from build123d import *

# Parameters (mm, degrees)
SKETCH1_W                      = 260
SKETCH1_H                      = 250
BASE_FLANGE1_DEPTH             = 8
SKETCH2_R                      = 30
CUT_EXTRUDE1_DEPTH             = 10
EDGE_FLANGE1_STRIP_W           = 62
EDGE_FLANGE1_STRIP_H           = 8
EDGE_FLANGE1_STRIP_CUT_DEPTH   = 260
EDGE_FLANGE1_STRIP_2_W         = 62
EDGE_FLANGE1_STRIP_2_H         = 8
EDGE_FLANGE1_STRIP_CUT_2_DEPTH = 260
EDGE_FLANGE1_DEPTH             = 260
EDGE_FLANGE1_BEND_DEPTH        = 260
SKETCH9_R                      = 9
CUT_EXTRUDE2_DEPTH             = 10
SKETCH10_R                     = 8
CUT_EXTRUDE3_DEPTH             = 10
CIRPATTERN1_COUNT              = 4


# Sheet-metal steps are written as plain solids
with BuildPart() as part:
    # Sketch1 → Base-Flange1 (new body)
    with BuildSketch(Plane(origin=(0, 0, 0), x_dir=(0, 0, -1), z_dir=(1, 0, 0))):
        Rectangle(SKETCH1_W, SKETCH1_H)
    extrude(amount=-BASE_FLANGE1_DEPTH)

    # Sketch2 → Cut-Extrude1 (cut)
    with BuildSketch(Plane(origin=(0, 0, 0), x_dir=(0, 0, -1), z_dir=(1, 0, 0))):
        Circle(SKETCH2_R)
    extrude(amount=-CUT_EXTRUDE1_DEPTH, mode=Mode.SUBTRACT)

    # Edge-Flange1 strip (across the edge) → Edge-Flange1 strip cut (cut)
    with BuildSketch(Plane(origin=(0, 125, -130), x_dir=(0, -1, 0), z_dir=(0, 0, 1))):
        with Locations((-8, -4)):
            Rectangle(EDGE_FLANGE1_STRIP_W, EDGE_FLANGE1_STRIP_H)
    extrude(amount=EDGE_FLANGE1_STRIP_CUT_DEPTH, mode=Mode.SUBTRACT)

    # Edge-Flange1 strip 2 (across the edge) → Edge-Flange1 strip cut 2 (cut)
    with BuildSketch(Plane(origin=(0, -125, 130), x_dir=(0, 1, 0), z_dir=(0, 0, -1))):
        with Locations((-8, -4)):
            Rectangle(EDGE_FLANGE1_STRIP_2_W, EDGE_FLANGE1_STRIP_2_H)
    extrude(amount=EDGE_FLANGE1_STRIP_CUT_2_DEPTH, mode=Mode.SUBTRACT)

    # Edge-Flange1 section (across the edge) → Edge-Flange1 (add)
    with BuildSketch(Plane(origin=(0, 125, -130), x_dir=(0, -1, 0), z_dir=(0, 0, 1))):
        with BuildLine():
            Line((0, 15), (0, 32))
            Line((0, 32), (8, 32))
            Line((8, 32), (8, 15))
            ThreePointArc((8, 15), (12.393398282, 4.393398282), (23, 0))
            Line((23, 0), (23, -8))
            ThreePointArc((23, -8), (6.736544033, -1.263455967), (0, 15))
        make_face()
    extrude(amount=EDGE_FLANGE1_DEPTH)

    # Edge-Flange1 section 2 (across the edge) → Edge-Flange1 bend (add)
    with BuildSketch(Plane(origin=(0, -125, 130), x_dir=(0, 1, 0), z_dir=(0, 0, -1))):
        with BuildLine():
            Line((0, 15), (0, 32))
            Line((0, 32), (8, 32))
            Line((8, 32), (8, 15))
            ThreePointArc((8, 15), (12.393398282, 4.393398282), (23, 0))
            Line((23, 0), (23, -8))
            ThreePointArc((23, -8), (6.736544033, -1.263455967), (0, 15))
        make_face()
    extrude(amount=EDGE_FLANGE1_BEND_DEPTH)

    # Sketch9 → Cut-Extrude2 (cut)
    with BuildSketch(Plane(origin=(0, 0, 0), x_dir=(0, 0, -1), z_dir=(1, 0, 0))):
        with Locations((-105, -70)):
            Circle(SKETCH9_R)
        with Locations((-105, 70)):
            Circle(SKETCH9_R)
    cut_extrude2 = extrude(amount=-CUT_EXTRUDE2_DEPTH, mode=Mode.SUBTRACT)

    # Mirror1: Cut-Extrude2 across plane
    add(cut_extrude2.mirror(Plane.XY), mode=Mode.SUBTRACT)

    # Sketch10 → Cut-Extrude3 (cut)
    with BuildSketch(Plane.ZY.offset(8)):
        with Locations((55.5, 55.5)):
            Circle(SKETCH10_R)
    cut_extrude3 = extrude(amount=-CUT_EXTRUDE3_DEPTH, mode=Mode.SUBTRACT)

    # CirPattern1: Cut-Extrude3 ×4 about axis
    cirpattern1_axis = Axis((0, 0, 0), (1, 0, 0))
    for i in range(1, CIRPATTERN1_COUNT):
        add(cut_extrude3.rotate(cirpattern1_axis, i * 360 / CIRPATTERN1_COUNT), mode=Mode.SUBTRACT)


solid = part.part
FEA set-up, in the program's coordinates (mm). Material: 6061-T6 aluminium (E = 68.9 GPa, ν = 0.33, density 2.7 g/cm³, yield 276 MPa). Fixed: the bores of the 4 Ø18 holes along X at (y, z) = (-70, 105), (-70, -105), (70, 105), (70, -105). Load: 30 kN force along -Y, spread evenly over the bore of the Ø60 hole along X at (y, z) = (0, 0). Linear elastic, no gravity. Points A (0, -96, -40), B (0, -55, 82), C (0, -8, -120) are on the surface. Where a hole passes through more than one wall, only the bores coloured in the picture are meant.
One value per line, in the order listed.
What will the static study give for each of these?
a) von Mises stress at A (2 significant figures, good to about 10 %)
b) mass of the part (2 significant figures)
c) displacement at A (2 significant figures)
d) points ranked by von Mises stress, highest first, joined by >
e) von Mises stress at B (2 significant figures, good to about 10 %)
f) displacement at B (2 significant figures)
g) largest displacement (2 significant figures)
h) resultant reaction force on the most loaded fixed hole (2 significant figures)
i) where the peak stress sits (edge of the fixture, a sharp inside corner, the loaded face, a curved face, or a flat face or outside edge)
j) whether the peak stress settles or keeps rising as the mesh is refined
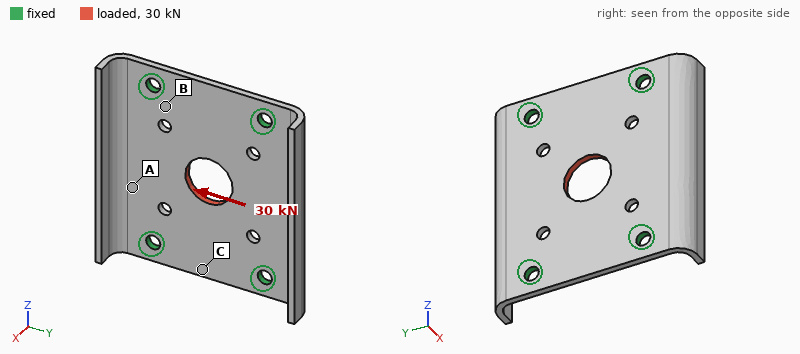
10 MPa
1.6 kg
38 µm
B > A > C
25 MPa
10 µm
61 µm
8.0 kN
edge of the fixture
keeps rising
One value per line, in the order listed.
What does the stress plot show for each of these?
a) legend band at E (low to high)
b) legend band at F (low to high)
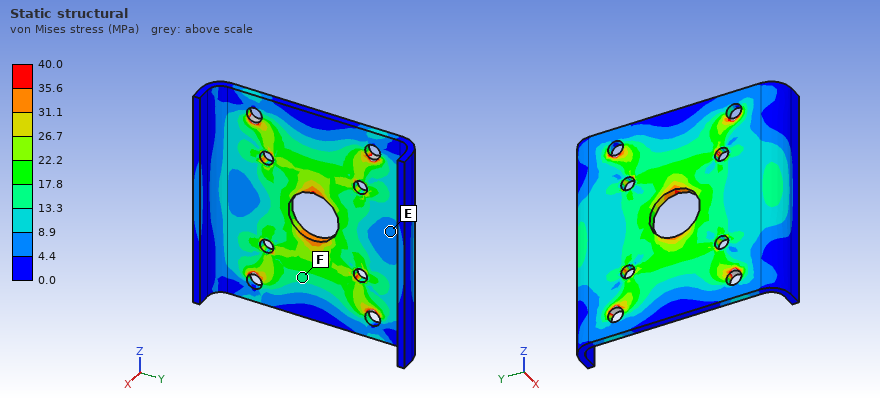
4.4 to 8.9 MPa
13.3 to 17.8 MPa
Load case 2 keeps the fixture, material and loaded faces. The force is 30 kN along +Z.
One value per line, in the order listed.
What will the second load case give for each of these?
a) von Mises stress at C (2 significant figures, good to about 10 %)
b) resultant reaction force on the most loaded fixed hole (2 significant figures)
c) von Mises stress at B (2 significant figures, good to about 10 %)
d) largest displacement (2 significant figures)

6.6 MPa
8.0 kN
22 MPa
29 µm
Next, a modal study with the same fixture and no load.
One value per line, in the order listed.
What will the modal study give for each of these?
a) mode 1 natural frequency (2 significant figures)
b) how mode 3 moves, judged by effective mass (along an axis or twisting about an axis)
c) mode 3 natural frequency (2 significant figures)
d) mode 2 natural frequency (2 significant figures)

1000 Hz
along X
1100 Hz
1100 Hz
